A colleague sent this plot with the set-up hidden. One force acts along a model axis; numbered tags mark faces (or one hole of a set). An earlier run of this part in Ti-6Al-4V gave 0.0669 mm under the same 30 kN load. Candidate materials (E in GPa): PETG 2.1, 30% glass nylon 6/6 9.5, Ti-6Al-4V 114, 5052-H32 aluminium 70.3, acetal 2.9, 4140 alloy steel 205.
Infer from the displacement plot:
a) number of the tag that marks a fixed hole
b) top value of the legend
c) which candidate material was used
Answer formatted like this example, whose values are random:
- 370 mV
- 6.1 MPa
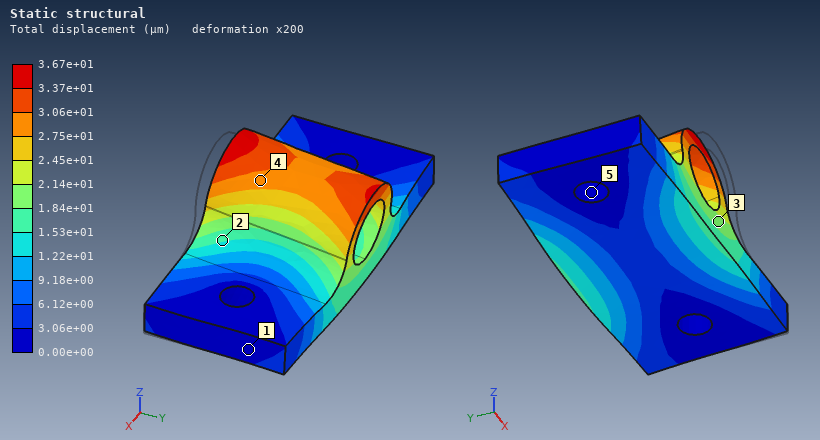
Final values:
- 5
- 3.67e+01 µm
- 4140 alloy steel
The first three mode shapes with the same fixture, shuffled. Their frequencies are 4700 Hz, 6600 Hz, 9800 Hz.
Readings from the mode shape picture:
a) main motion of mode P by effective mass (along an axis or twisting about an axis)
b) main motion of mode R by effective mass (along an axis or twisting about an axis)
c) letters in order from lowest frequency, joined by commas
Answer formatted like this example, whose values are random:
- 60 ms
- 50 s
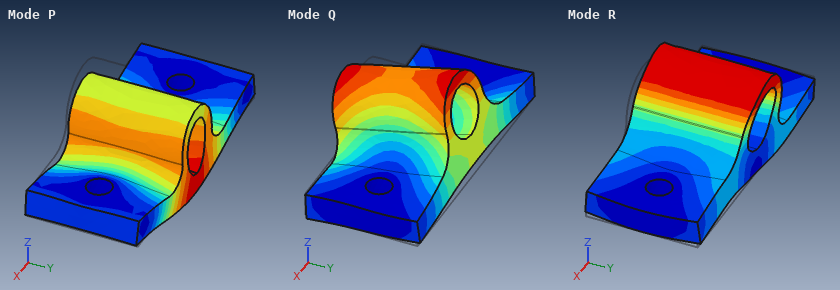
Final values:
- along Z
- along X
- Q, P, R
